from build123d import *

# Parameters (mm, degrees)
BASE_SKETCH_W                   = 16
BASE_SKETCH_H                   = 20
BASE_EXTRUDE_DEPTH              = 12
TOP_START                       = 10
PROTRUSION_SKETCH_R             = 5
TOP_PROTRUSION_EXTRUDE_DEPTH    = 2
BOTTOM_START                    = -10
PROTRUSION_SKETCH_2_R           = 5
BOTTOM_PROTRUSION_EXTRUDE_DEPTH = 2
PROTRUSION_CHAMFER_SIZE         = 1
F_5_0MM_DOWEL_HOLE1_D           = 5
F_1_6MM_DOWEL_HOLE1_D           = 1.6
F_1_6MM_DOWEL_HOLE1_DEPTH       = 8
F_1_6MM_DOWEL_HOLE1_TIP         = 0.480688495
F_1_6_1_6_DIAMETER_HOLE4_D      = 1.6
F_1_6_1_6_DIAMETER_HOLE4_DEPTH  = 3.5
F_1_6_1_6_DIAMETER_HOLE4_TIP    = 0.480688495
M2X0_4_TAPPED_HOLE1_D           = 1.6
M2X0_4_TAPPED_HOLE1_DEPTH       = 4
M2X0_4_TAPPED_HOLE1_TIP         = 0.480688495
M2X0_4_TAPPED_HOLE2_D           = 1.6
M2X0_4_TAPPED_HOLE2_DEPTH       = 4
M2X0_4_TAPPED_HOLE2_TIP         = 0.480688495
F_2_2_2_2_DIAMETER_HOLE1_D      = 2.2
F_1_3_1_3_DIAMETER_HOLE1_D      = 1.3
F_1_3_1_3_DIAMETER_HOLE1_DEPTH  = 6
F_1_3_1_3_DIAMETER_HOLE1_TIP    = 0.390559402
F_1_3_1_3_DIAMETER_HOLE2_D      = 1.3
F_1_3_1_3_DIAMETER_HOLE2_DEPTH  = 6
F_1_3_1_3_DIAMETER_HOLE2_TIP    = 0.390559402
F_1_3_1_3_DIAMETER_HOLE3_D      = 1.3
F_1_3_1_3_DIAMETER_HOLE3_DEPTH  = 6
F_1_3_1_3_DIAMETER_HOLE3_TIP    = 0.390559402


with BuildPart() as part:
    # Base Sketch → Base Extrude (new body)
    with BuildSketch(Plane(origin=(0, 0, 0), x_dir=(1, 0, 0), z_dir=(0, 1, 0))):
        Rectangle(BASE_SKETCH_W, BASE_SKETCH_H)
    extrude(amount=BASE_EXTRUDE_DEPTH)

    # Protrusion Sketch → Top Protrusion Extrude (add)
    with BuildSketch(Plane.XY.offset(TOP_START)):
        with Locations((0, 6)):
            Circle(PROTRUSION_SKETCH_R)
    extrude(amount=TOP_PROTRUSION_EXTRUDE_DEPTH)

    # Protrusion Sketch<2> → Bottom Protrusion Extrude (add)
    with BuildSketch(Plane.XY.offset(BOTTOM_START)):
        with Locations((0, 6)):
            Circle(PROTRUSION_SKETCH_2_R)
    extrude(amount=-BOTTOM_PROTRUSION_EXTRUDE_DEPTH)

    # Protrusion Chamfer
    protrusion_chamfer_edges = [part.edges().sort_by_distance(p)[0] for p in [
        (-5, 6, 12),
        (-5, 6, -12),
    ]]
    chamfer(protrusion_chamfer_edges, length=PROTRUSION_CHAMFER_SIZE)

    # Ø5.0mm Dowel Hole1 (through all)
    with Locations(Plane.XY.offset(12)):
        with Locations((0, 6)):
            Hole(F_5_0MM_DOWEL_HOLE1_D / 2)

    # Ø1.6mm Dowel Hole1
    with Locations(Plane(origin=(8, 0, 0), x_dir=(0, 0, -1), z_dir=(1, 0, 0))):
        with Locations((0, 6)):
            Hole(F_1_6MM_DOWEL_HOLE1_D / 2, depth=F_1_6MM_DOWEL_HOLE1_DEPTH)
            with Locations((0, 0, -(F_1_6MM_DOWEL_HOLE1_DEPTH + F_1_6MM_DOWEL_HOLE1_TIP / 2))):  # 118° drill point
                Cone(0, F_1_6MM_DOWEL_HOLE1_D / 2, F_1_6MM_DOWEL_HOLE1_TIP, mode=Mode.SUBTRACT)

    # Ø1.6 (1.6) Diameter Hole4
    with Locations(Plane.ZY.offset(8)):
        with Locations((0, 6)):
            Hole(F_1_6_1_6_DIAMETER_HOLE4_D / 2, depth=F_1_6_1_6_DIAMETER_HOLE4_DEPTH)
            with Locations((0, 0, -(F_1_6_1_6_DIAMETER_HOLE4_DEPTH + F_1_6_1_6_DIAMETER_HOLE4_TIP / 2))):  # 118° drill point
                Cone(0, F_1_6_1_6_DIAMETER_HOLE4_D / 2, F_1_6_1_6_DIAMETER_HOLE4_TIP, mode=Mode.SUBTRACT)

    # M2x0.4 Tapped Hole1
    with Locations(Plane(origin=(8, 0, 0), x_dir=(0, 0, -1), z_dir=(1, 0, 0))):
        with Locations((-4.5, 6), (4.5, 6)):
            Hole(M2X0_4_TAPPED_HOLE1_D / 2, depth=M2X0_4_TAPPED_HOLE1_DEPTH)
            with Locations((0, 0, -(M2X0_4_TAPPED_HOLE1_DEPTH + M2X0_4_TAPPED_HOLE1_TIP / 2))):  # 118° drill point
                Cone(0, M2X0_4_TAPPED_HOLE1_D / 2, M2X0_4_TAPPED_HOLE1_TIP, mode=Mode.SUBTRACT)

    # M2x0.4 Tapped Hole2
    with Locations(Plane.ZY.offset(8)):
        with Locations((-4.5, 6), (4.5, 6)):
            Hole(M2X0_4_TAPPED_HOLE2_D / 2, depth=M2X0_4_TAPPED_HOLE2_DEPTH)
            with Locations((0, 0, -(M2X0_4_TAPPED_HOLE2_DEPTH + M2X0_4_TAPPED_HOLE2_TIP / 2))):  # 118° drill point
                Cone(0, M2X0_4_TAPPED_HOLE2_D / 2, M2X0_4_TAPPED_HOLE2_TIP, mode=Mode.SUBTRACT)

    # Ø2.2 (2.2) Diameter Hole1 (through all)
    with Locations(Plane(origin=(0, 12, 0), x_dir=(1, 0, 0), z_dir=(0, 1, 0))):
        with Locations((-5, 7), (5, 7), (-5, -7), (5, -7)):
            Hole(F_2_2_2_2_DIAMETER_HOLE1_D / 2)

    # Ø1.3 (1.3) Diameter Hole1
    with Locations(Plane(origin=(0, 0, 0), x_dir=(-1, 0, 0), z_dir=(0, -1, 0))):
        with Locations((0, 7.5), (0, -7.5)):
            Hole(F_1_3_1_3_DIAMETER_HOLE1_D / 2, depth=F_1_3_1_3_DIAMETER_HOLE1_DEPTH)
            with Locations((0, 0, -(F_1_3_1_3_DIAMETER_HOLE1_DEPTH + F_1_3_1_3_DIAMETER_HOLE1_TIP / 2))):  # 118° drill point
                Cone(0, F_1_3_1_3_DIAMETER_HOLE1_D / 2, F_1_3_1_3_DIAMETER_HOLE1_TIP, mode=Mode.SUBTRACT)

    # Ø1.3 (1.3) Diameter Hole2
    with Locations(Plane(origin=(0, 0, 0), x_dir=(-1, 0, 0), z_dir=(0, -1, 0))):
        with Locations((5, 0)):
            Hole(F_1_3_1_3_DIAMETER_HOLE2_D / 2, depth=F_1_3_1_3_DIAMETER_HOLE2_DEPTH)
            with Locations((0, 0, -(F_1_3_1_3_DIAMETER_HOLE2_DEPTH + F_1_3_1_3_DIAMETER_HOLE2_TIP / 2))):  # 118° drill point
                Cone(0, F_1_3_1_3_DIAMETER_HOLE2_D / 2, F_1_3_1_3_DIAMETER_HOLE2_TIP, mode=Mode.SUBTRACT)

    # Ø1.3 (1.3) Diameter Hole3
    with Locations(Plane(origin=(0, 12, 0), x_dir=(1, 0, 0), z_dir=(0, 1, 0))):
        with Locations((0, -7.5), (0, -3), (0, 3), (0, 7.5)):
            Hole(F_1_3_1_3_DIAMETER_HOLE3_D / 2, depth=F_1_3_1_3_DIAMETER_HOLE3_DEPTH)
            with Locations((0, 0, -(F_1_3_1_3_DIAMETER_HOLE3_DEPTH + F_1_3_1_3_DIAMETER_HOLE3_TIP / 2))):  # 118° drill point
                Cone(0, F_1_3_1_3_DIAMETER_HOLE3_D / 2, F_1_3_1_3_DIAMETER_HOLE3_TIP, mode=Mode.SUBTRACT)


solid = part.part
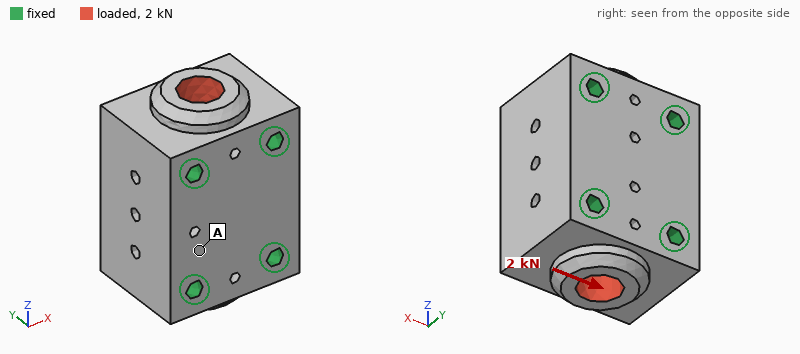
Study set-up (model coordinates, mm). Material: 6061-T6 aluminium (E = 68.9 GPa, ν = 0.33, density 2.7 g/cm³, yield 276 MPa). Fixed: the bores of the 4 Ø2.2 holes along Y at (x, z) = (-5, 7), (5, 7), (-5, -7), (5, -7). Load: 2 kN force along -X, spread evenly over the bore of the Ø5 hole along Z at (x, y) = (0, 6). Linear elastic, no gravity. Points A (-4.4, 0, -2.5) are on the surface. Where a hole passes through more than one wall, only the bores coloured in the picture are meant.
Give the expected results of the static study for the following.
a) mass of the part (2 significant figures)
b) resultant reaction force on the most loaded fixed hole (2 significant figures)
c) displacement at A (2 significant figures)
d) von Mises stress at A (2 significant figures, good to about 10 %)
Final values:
9.1 g
500 N
0.43 µm
2.4 MPa
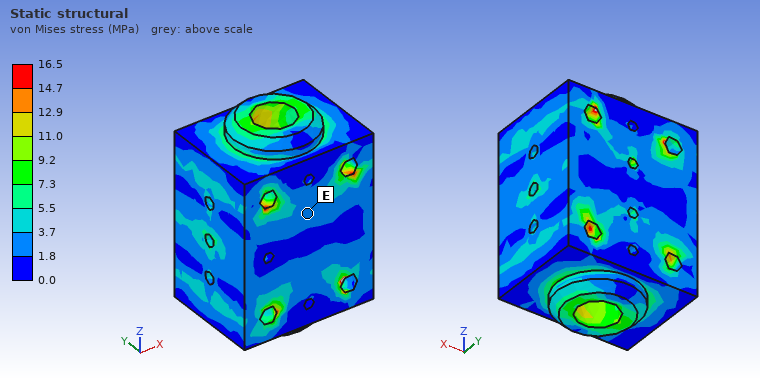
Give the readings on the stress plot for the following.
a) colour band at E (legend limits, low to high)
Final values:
1.8 to 3.7 MPa
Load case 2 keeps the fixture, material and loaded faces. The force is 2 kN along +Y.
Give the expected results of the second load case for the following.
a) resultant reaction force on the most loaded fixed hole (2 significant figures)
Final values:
500 N
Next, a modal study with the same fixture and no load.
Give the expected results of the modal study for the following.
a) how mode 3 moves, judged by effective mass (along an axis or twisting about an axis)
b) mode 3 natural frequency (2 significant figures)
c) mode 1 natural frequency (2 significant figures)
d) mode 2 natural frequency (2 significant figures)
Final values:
twisting about Z
110 kHz
95 kHz
99 kHz
